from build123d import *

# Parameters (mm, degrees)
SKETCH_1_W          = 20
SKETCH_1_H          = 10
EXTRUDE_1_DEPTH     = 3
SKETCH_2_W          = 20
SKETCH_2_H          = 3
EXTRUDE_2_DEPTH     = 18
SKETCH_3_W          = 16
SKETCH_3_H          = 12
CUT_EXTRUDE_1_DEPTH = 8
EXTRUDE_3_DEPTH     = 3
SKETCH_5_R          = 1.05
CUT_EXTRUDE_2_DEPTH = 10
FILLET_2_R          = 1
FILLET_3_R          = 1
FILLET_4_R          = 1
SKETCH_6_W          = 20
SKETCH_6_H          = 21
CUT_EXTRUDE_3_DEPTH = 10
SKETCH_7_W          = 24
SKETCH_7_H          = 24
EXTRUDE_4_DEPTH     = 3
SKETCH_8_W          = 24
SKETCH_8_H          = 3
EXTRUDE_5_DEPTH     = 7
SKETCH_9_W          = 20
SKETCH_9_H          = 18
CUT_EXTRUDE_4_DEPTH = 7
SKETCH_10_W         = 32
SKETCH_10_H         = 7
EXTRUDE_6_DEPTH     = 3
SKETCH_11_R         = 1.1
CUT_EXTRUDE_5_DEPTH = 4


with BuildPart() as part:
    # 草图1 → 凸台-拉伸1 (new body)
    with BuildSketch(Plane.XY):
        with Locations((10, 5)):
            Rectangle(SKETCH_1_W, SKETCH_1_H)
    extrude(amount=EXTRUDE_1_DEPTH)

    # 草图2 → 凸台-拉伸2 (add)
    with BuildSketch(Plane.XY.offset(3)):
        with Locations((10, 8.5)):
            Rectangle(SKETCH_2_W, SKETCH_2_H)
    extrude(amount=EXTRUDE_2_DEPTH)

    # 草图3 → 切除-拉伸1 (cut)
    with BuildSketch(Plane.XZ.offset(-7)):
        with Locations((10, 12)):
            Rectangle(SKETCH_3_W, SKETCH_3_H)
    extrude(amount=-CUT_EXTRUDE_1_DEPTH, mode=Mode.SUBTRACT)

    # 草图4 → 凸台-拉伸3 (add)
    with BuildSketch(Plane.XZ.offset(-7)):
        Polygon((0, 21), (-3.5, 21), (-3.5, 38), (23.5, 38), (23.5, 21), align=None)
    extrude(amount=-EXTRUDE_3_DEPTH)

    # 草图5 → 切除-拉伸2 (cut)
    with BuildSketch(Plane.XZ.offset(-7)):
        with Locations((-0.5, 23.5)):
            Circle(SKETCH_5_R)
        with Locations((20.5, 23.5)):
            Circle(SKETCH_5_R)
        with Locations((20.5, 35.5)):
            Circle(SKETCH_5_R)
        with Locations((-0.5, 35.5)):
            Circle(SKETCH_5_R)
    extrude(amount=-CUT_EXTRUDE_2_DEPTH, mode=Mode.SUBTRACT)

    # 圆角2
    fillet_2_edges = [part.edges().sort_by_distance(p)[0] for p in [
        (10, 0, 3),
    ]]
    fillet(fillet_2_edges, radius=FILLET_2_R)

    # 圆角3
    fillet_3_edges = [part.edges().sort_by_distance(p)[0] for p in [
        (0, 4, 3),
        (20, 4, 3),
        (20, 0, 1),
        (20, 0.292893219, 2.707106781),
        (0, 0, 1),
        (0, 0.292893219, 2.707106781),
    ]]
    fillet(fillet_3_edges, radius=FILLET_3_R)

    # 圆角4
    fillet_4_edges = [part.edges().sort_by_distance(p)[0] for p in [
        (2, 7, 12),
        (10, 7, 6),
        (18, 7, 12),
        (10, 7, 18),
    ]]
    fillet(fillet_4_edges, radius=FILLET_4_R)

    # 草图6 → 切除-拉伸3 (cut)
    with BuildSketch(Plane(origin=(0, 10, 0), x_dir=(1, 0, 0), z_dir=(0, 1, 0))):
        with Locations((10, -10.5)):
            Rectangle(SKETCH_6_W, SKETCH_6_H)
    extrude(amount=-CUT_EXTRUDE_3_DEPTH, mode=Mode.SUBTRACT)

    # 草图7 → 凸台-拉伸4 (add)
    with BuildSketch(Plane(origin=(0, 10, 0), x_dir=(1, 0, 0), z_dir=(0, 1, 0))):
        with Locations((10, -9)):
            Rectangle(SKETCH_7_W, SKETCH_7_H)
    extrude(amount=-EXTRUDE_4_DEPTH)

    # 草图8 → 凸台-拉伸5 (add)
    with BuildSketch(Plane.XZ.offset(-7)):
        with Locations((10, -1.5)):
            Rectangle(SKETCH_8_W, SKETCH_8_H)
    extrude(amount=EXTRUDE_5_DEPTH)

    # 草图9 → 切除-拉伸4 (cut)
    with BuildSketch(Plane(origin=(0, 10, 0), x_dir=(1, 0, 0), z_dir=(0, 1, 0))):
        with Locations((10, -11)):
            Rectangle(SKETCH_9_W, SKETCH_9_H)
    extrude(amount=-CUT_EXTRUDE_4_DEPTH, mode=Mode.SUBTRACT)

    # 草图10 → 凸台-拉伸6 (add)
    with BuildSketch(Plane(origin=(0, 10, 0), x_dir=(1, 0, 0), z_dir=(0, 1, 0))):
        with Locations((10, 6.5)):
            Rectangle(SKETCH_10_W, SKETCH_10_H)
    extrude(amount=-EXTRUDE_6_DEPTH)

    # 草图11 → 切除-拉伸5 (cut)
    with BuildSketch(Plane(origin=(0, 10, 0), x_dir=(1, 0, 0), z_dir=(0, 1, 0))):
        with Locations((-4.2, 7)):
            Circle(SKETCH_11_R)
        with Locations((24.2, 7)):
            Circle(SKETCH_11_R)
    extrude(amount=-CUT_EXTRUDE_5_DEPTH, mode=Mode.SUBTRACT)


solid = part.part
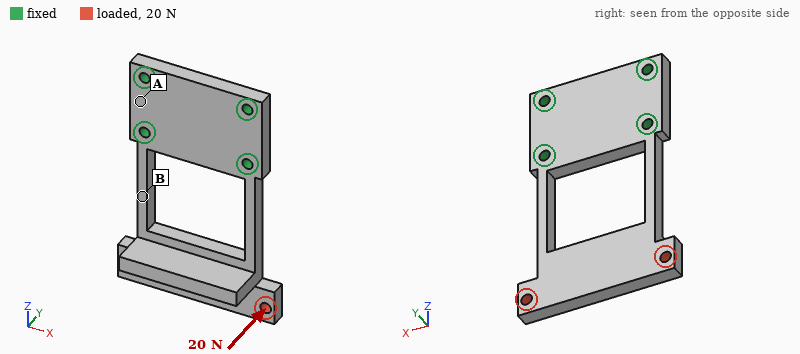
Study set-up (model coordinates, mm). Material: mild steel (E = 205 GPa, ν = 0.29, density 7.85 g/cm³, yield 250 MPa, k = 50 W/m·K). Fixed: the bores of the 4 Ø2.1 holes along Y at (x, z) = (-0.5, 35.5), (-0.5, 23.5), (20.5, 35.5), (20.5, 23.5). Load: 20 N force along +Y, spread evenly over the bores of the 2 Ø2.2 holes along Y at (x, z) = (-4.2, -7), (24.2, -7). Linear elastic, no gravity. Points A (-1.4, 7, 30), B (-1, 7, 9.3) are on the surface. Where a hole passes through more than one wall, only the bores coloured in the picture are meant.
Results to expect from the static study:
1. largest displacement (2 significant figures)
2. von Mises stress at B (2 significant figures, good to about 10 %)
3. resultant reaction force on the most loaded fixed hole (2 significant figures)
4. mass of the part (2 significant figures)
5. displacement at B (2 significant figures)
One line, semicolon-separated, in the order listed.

100 µm; 54 MPa; 13 N; 25 g; 22 µm
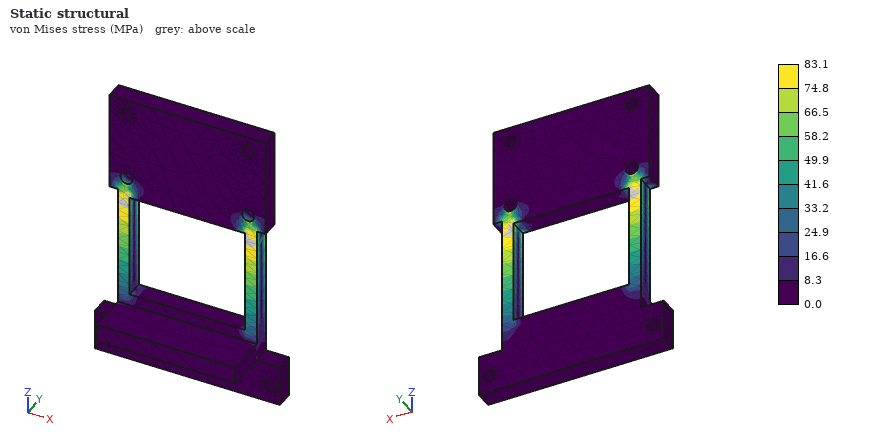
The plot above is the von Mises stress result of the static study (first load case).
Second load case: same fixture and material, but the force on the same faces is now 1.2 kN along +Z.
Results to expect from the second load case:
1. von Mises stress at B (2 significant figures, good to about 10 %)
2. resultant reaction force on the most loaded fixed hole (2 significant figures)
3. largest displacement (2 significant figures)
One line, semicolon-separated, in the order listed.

100 MPa; 580 N; 18 µm
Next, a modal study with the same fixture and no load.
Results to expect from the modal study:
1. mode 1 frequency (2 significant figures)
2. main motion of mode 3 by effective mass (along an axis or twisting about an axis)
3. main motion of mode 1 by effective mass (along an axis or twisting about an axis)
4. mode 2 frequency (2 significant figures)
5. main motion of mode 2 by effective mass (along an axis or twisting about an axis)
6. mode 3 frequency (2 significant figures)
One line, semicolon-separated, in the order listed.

820 Hz; twisting about Z; along Y; 1500 Hz; along X; 2700 Hz
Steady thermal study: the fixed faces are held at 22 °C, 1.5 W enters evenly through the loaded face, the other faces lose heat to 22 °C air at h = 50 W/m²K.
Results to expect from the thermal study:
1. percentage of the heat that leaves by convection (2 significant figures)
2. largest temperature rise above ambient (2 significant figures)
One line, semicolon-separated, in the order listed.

76 %; 20 K
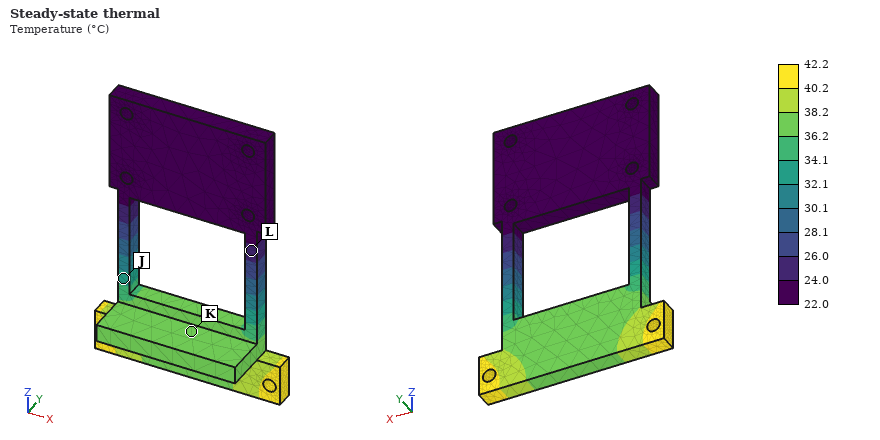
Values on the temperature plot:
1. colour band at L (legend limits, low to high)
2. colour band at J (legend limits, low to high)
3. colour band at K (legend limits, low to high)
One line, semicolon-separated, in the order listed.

24.0 to 26.0 °C; 32.1 to 34.1 °C; 36.2 to 38.2 °C
